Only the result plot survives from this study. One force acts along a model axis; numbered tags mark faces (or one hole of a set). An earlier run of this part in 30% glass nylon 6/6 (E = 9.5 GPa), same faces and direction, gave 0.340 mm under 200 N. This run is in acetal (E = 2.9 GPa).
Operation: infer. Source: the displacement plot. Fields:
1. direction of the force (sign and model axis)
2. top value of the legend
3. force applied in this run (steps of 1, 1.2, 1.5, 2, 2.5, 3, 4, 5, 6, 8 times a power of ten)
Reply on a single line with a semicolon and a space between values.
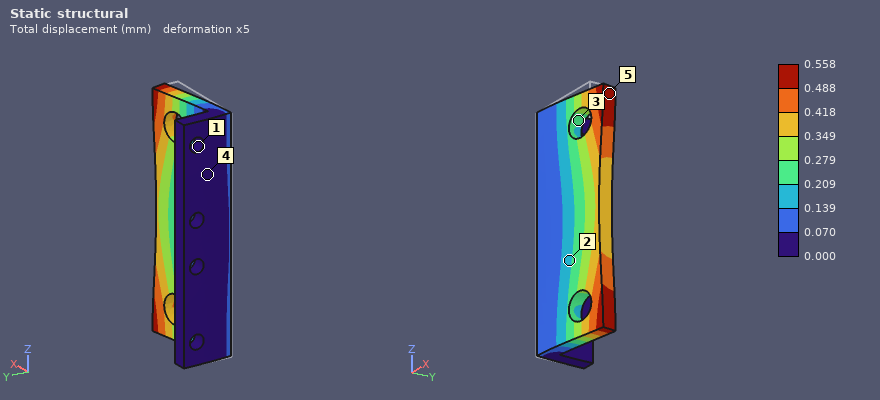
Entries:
+Y; 0.558 mm; 100 N
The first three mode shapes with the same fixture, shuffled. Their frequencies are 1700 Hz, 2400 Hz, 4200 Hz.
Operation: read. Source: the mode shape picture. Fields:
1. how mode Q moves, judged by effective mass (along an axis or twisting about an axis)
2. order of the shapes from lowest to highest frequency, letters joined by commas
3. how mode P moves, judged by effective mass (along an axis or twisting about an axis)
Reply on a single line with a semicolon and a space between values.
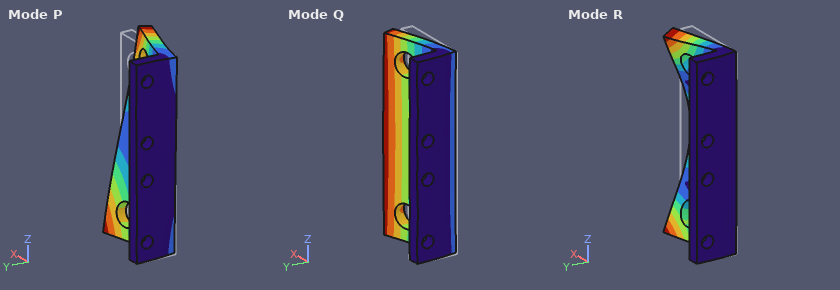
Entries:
along Y; Q, P, R; twisting about X
